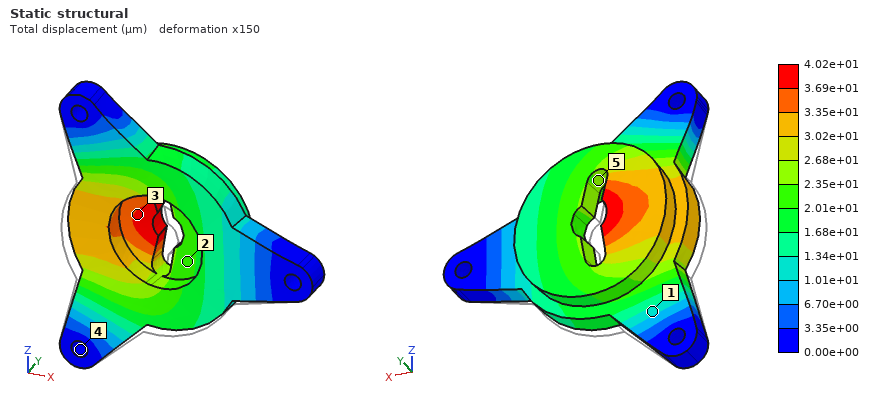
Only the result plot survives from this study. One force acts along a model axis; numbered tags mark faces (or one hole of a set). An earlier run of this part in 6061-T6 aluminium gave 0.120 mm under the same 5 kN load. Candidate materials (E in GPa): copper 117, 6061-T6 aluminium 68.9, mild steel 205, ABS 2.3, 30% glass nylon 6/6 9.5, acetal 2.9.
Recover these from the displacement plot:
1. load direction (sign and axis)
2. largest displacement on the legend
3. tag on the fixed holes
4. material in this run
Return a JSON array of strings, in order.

["+Y", "4.02e+01 µm", "4", "mild steel"]
